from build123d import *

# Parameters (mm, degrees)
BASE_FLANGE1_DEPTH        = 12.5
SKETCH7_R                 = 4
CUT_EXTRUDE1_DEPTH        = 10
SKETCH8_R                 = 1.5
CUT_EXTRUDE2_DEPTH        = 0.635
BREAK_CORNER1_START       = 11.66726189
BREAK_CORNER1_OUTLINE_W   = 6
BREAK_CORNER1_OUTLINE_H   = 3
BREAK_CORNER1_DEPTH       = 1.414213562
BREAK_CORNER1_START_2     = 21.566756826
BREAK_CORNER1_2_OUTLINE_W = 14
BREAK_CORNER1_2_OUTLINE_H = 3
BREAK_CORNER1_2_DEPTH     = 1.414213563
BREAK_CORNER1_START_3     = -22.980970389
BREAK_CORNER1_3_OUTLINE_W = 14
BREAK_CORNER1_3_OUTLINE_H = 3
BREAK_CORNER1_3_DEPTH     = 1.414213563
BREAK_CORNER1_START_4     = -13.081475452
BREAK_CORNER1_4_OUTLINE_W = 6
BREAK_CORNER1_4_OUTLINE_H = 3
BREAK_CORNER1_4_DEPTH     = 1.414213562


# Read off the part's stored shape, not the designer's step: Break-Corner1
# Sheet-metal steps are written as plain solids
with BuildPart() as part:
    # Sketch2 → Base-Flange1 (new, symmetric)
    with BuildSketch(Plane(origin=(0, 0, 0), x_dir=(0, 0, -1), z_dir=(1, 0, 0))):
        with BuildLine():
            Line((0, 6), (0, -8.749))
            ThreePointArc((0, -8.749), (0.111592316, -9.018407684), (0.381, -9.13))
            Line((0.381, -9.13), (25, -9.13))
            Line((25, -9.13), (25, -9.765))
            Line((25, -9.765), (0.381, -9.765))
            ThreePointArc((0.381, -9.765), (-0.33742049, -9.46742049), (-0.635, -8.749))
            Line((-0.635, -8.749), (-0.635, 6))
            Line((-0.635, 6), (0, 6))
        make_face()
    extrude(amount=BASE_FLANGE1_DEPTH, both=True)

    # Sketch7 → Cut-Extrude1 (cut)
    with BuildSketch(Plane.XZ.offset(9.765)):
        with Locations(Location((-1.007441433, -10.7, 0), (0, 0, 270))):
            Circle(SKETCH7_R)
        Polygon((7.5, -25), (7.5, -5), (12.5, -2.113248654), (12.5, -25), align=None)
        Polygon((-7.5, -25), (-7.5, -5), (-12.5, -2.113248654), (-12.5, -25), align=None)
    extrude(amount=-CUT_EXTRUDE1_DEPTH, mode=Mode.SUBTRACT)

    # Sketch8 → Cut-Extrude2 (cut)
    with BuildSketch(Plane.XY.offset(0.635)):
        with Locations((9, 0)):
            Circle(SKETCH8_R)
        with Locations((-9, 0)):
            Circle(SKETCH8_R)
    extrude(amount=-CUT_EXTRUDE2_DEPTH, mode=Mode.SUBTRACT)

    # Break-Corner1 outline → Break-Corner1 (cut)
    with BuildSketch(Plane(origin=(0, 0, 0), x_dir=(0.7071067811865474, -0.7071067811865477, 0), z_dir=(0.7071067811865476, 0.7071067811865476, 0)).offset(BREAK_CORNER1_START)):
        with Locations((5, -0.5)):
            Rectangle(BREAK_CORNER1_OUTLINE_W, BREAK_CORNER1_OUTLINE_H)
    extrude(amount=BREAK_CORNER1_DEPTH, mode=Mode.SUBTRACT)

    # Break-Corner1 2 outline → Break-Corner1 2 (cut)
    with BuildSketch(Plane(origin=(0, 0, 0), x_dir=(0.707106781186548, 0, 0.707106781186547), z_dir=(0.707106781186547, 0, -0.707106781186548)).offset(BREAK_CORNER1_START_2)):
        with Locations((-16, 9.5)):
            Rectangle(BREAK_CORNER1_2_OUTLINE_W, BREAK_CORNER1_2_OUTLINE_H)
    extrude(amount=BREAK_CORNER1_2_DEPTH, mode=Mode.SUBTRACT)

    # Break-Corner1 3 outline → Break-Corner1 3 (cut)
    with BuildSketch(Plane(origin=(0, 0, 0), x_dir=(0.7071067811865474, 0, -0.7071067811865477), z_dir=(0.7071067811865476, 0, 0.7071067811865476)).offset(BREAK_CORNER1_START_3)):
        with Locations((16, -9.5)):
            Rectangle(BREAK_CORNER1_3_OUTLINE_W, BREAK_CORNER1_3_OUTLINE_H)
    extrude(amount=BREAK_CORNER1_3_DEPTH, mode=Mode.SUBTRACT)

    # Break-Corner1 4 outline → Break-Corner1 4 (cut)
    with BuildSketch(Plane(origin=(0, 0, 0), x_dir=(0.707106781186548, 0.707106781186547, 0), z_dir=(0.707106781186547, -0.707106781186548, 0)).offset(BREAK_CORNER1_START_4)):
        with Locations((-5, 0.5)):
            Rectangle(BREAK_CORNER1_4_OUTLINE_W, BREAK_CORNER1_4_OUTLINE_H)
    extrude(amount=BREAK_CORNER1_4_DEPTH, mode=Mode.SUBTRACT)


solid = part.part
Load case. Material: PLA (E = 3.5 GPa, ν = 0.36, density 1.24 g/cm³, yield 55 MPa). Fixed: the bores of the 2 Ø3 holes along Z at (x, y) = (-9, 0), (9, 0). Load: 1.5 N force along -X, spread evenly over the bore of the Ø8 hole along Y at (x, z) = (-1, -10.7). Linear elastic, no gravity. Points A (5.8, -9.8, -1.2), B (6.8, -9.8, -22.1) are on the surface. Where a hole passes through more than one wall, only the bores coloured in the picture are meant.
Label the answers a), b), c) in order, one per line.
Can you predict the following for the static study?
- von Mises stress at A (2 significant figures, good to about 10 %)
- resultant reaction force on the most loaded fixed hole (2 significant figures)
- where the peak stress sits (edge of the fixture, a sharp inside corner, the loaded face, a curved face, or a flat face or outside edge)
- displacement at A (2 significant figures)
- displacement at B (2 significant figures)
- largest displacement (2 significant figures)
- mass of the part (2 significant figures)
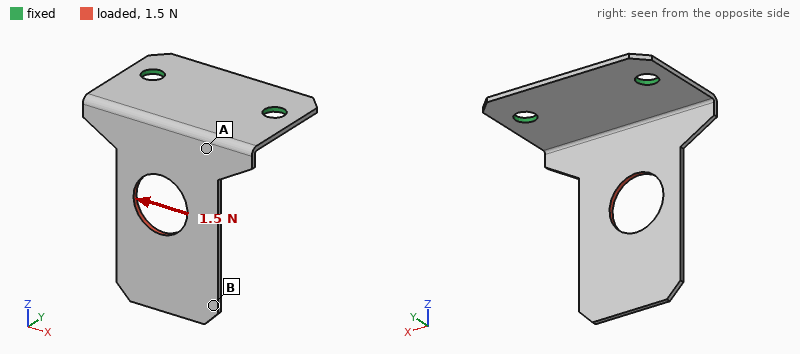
a) 2.7 MPa
b) 1.3 N
c) a flat face or outside edge
d) 0.086 mm
e) 0.34 mm
f) 0.37 mm
g) 0.57 g
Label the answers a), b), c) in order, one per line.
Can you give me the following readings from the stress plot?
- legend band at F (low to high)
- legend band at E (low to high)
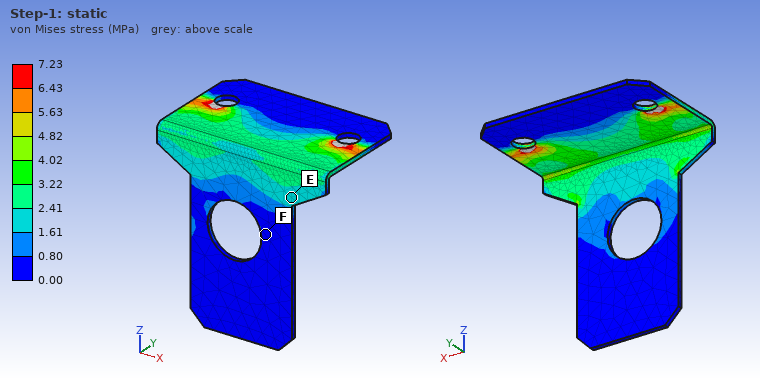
a) 0.00 to 0.80 MPa
b) 1.61 to 2.41 MPa
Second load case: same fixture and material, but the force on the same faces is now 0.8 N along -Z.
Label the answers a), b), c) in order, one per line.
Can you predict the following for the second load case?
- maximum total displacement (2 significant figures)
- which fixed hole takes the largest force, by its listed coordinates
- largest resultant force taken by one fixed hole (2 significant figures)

a) 0.40 mm
b) (-9, 0)
c) 0.44 N
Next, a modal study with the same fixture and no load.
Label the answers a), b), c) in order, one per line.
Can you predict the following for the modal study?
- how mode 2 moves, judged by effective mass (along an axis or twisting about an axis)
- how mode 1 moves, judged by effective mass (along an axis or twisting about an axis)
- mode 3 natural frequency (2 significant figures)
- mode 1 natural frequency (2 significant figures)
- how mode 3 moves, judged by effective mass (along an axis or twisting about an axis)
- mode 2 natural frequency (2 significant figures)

a) along X
b) along Y
c) 880 Hz
d) 210 Hz
e) along Z
f) 640 Hz
